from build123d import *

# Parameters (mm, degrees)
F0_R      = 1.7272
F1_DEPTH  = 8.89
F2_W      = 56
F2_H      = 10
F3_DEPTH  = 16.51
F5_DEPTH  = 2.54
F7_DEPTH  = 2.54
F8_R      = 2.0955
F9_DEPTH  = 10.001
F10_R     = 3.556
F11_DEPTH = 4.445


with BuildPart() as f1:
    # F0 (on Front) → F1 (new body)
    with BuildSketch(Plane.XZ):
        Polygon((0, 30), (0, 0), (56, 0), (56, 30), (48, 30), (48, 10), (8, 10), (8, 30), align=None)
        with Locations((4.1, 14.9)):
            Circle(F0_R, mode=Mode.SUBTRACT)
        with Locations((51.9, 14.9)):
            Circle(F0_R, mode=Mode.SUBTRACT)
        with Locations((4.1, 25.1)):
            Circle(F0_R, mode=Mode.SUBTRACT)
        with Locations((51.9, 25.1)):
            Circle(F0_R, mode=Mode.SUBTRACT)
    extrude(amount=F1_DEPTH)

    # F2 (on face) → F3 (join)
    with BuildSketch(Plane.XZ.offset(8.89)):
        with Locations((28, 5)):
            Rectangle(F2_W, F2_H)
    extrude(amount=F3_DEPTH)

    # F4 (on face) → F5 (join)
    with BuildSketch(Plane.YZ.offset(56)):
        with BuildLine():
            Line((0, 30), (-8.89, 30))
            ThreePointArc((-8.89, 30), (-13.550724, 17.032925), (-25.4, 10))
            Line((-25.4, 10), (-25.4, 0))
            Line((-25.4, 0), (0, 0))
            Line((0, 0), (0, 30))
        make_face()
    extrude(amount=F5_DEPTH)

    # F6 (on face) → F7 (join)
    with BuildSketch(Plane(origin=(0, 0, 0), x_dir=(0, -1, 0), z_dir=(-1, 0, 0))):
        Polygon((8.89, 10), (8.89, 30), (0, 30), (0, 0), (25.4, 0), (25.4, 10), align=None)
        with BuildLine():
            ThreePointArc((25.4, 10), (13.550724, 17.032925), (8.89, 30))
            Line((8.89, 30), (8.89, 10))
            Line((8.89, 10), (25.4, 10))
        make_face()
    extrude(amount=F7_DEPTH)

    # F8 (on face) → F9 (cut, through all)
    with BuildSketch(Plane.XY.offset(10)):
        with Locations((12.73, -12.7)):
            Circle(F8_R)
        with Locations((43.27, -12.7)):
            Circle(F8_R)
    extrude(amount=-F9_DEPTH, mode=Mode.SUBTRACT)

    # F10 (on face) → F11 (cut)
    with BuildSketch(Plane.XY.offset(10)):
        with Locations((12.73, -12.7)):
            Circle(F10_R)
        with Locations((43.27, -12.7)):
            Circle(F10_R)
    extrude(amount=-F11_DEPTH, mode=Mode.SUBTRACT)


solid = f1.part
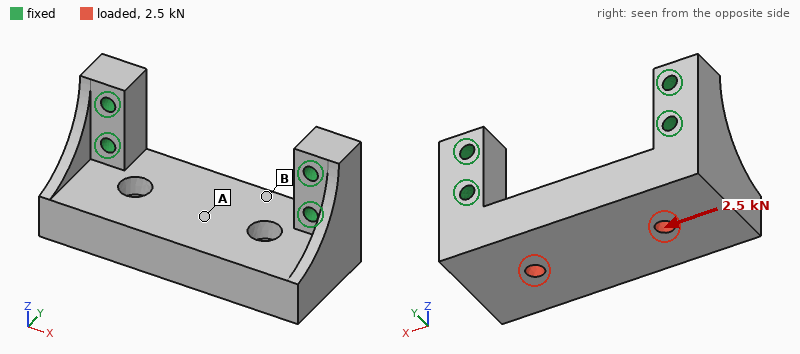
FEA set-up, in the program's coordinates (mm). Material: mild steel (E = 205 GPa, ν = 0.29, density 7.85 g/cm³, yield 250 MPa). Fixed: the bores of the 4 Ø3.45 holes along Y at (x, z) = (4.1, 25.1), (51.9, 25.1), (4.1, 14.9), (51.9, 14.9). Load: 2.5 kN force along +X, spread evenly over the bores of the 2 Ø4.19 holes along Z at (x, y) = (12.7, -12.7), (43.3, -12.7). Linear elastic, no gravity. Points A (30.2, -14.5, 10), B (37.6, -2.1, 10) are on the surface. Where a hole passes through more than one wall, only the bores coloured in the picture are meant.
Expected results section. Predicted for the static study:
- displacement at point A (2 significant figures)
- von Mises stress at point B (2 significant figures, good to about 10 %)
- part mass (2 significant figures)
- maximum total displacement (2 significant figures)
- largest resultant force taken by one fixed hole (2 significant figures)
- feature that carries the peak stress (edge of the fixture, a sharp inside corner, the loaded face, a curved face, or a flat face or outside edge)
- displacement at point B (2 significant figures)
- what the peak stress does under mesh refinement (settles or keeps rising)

3.6 µm
14 MPa
150 g
4.2 µm
1.6 kN
edge of the fixture
2.9 µm
keeps rising
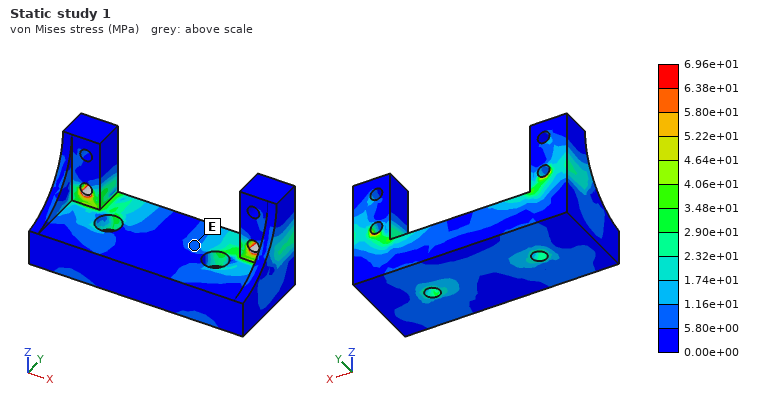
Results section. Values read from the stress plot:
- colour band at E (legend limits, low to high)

5.80e+00 to 1.16e+01 MPa
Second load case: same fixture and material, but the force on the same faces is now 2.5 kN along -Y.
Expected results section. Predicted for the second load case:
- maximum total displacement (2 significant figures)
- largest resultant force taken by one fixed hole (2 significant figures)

14 µm
1.6 kN
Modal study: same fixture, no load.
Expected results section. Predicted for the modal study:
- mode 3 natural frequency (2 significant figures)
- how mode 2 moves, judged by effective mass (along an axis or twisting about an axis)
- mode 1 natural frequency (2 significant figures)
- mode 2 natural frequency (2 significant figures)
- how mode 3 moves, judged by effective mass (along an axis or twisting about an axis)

14 kHz
along X
6700 Hz
12 kHz
along Y
